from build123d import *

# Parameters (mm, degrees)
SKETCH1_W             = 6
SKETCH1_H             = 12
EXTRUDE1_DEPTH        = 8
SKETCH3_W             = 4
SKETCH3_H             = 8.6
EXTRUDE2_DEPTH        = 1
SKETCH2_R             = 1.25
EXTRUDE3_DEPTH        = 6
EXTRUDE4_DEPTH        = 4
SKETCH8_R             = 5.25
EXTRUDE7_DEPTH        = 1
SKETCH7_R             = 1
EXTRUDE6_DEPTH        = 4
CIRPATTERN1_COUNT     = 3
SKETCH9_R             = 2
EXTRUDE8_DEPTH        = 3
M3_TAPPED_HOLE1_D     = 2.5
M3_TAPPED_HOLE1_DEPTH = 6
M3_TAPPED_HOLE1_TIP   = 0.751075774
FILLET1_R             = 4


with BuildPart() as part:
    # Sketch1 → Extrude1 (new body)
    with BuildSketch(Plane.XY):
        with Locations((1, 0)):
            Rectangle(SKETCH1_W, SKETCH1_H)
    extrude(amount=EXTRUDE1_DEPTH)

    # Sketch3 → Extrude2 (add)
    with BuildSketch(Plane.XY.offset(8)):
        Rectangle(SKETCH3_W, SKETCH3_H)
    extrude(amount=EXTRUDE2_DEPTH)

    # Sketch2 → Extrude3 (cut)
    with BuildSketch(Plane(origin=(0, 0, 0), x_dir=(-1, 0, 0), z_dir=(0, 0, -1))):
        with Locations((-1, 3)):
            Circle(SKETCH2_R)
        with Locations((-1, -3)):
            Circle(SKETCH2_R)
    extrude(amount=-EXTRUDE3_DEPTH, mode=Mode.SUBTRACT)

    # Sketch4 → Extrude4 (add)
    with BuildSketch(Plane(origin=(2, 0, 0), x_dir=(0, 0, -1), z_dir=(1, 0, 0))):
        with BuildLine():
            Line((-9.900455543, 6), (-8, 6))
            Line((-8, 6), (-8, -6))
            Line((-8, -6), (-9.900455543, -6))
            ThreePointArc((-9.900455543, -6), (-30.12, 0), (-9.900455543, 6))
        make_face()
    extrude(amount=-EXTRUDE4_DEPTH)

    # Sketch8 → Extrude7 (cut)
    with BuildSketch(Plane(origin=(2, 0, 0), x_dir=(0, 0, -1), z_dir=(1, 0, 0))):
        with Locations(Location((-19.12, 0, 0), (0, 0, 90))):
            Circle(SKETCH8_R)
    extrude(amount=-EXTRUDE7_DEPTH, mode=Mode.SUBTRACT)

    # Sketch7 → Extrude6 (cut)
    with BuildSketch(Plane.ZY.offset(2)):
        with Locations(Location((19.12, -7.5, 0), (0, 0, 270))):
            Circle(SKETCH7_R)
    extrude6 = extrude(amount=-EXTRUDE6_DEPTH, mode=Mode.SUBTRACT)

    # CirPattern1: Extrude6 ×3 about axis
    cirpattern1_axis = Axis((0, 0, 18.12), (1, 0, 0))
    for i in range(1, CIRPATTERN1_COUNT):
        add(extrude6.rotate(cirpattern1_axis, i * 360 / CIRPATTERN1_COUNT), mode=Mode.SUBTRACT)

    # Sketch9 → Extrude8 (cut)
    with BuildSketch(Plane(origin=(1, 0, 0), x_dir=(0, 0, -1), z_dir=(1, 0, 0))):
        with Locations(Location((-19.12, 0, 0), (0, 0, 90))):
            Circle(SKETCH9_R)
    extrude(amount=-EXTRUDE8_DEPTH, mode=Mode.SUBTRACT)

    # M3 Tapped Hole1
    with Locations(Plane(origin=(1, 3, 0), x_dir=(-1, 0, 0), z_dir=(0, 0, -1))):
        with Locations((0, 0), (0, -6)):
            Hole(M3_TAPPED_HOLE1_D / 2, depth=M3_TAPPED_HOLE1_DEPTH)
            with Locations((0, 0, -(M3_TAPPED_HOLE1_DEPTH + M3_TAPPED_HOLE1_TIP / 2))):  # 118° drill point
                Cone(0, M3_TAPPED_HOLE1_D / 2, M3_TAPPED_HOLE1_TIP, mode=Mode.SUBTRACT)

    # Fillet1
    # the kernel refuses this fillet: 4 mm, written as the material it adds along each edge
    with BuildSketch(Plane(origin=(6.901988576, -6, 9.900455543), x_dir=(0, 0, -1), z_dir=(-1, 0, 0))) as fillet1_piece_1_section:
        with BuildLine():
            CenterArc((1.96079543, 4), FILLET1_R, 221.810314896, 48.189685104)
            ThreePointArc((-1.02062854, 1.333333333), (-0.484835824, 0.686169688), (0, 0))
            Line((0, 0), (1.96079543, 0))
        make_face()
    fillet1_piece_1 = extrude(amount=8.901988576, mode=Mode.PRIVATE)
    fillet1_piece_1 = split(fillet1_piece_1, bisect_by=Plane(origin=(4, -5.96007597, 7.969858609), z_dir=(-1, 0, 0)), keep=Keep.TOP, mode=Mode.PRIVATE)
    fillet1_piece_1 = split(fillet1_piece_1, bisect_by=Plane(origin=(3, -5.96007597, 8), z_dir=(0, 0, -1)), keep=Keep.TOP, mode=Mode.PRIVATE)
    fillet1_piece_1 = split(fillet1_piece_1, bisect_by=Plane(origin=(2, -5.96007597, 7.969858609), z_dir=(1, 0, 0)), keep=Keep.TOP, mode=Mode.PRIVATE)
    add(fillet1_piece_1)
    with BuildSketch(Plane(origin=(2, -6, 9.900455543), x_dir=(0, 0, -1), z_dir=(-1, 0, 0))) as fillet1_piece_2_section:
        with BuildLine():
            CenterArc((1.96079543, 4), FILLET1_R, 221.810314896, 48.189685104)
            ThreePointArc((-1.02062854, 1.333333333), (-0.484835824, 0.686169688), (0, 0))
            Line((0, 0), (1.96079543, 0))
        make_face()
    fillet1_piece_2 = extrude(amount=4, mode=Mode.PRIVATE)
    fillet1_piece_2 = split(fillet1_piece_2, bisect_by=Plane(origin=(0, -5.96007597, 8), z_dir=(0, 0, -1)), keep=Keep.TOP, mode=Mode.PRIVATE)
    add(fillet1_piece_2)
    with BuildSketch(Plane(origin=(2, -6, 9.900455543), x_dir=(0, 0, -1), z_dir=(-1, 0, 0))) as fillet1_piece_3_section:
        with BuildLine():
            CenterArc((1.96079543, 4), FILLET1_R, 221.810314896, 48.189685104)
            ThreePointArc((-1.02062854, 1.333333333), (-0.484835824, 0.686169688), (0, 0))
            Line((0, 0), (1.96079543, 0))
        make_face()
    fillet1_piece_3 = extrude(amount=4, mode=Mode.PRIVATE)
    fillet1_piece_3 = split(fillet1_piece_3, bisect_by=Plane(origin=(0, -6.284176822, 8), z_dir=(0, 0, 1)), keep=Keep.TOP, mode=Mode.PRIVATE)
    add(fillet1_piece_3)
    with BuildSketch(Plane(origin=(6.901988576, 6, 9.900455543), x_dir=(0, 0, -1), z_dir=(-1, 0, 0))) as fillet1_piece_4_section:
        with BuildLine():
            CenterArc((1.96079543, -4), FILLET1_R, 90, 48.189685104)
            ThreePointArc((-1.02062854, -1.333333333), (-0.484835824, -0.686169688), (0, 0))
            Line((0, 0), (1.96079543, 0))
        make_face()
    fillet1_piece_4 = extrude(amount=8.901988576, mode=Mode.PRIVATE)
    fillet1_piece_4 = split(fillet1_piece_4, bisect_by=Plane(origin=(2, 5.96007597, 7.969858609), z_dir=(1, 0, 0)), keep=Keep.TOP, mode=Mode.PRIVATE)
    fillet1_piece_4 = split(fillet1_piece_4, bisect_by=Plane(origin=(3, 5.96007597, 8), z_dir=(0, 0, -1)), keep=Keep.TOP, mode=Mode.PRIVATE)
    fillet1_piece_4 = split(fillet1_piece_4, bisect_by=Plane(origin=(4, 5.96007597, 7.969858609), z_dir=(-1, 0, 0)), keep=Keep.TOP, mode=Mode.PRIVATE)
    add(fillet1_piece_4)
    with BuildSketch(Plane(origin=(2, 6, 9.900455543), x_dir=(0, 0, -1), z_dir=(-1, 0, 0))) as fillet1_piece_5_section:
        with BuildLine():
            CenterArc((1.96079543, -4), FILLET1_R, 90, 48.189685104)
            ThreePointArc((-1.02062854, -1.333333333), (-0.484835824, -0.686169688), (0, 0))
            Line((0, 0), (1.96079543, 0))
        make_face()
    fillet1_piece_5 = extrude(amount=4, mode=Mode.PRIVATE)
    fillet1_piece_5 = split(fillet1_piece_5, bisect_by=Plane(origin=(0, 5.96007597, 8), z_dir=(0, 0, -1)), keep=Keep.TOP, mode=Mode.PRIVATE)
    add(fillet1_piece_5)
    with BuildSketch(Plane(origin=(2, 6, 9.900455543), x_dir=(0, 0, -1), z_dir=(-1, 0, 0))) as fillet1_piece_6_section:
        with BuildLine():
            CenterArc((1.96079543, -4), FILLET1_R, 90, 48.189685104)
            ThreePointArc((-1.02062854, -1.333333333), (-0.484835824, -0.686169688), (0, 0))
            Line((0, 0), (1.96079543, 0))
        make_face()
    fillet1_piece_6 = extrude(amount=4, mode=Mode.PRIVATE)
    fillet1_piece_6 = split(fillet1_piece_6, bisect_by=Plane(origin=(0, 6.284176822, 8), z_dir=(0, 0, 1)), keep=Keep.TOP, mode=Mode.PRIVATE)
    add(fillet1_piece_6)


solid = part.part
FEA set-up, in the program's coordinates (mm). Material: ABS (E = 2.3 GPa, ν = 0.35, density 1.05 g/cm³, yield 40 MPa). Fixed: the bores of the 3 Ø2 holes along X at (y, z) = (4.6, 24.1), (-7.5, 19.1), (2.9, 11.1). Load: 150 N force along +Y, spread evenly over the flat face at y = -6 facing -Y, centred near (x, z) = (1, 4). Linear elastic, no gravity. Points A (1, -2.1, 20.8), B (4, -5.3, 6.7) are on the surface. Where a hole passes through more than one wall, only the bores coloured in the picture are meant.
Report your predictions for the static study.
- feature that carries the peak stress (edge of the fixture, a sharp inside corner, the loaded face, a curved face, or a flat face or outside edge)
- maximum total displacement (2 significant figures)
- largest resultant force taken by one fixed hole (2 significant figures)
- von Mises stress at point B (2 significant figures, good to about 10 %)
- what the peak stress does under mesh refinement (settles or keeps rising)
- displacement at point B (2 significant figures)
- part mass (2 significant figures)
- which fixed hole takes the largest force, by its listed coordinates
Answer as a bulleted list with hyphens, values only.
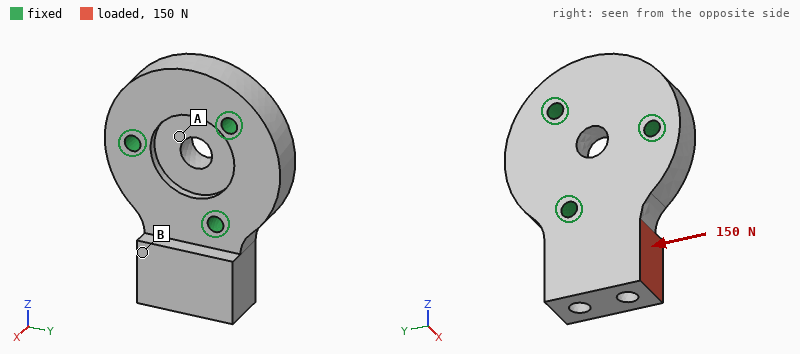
- edge of the fixture
- 96 µm
- 160 N
- 3.3 MPa
- keeps rising
- 58 µm
- 2.0 g
- (2.9, 11.1)
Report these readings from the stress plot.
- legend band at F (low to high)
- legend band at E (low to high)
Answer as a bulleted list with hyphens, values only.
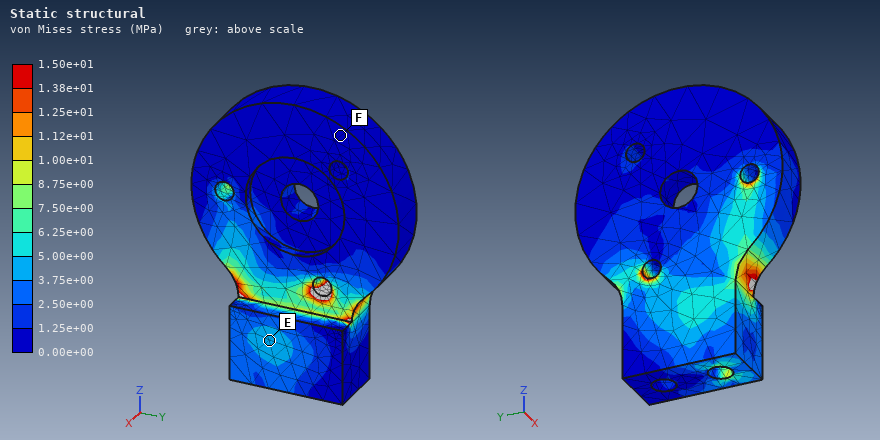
- 0.00e+00 to 1.25e+00 MPa
- 3.75e+00 to 5.00e+00 MPa
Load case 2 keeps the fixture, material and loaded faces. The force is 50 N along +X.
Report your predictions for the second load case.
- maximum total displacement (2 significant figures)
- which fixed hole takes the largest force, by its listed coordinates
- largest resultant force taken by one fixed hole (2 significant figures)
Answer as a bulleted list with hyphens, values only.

- 0.23 mm
- (2.9, 11.1)
- 46 N
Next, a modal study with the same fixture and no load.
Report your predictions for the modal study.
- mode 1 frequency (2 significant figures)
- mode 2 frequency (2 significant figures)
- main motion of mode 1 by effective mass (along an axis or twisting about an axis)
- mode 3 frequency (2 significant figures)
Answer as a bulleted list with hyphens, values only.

- 5100 Hz
- 10000 Hz
- along X
- 11 kHz
